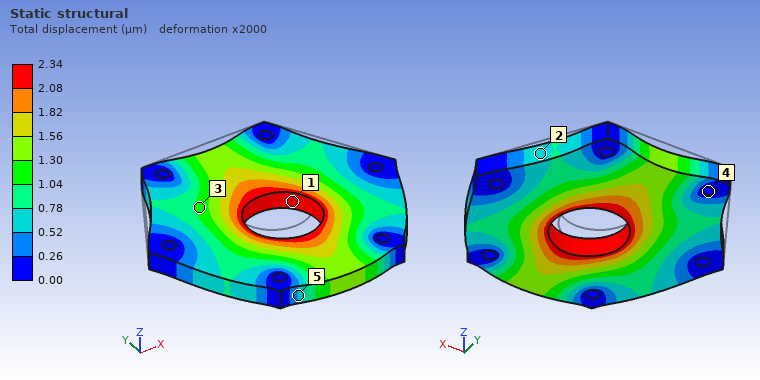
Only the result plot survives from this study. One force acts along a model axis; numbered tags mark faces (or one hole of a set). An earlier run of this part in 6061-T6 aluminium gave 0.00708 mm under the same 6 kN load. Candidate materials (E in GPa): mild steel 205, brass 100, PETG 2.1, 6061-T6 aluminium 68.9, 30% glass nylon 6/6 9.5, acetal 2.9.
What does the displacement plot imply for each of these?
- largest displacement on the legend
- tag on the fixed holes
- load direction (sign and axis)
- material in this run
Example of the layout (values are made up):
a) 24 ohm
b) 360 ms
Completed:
a) 2.34 µm
b) 4
c) -Y
d) mild steel
